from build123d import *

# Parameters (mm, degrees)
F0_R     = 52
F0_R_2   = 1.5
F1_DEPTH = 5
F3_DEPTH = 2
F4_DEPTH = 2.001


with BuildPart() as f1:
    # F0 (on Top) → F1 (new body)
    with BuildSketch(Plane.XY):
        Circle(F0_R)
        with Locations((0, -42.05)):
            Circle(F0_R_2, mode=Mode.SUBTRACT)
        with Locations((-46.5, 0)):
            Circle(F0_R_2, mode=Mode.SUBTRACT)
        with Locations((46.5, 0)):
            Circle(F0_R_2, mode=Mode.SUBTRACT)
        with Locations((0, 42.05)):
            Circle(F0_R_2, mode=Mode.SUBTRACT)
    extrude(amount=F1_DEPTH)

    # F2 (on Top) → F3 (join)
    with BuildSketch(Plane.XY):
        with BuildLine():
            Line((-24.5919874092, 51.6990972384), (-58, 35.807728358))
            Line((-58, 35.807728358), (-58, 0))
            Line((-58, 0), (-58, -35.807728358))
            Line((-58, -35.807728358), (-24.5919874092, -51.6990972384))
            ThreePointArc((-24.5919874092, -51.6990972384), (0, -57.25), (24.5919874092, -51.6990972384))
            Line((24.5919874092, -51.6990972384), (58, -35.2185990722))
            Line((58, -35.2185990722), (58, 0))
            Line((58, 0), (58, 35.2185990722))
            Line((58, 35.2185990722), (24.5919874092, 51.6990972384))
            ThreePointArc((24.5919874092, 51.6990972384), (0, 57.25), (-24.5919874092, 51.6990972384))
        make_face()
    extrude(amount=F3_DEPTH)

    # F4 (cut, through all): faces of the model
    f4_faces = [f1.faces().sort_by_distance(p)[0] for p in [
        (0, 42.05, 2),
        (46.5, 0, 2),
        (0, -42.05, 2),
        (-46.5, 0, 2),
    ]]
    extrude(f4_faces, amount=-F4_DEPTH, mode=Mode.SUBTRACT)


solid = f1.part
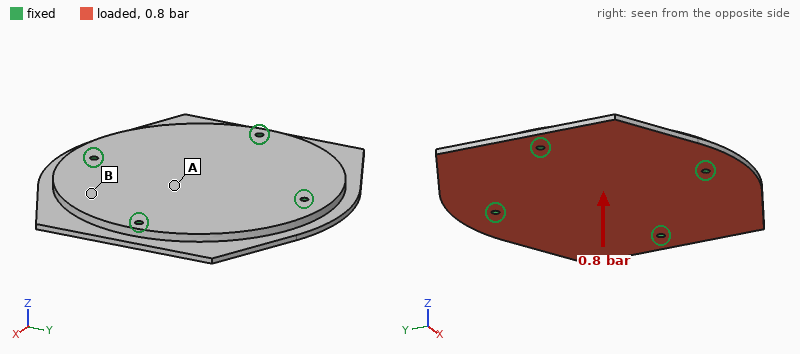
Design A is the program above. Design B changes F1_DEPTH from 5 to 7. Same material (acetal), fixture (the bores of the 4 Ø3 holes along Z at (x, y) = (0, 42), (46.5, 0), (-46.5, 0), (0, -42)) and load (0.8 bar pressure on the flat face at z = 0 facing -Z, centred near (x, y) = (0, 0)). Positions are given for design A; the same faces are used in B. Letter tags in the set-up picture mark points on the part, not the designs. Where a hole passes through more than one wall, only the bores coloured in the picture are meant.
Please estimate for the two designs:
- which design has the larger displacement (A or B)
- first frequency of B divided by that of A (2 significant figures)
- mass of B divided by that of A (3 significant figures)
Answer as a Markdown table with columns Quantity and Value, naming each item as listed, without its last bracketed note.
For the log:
| Quantity | Value |
|---|---|
| which design has the larger displacement | A |
| first frequency of B divided by that of A | 1.4 |
| mass of B divided by that of A | 1.35 |
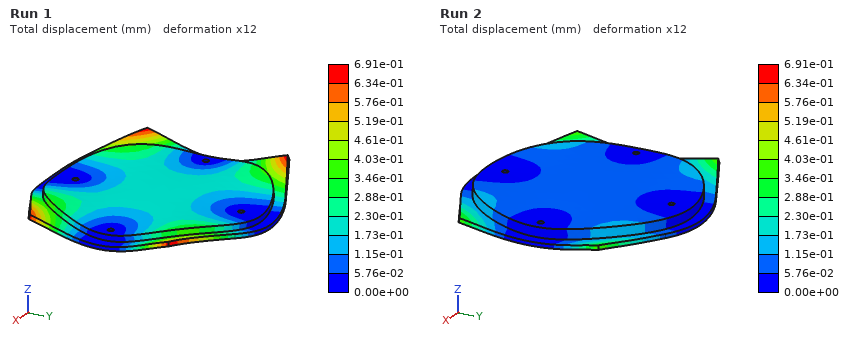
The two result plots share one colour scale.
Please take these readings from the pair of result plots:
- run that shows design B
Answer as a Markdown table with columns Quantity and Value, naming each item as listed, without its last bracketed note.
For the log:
| Quantity | Value |
|---|---|
| run that shows design B | Run 2 |
